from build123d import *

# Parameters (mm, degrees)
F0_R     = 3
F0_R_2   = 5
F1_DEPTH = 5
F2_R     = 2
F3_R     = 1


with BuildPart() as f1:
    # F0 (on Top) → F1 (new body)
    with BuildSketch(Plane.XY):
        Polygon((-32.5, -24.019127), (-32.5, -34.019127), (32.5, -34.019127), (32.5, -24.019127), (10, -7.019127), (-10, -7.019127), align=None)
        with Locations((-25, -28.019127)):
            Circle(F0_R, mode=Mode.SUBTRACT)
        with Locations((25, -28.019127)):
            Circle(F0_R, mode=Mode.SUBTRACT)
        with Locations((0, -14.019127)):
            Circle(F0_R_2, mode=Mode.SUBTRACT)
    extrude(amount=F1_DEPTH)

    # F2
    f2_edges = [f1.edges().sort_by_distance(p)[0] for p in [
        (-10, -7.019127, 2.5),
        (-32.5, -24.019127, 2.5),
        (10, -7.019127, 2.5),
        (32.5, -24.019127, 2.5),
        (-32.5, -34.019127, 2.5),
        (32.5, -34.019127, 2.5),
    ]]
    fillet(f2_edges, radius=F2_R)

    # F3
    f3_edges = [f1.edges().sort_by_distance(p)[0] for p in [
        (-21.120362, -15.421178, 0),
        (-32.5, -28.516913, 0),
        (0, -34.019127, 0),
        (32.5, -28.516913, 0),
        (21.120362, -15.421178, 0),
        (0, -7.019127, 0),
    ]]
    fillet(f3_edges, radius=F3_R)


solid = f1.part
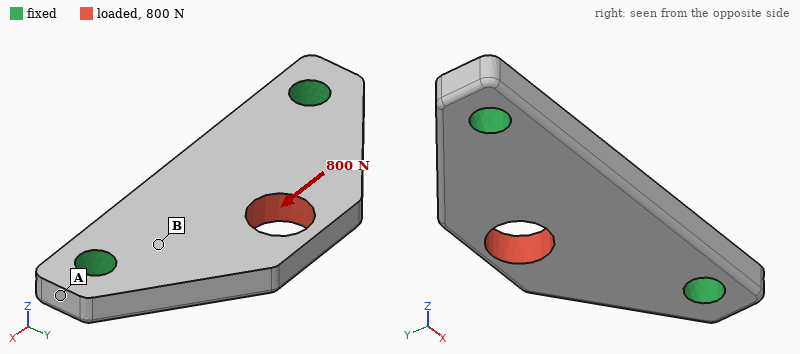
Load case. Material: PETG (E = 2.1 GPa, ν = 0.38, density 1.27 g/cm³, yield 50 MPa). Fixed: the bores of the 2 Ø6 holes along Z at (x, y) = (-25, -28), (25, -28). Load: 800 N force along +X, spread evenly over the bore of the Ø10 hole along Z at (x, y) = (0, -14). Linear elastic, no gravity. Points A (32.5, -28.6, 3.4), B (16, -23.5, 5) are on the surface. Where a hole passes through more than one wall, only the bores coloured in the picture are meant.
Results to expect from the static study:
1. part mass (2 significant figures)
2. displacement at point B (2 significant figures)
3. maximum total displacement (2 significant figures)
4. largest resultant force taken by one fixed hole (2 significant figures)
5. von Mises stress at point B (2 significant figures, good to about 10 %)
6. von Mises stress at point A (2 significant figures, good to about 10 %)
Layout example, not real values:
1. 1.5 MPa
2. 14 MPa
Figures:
1. 7.8 g
2. 0.025 mm
3. 0.14 mm
4. 450 N
5. 5.3 MPa
6. 2.2 MPa
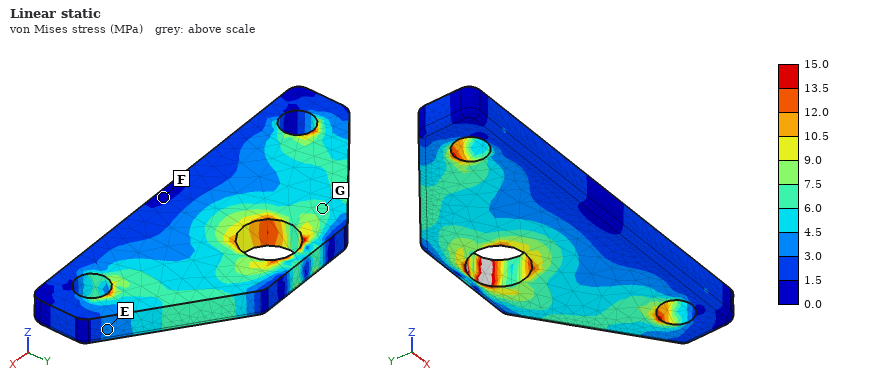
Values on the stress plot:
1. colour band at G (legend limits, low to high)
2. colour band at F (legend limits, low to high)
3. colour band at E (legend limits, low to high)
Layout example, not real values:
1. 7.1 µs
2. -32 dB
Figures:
1. 6.0 to 7.5 MPa
2. 0.0 to 1.5 MPa
3. 3.0 to 4.5 MPa
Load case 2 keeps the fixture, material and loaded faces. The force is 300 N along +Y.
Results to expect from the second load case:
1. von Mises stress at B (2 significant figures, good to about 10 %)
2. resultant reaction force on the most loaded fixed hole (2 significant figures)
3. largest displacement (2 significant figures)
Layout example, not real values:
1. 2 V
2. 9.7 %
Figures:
1. 3.3 MPa
2. 180 N
3. 86 µm
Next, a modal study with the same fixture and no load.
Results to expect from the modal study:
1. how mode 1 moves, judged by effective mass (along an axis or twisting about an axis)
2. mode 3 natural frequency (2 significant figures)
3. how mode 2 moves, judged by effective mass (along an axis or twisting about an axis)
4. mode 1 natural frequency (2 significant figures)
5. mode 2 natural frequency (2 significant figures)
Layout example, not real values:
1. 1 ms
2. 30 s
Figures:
1. along Z
2. 4400 Hz
3. along Z
4. 1800 Hz
5. 3300 Hz
